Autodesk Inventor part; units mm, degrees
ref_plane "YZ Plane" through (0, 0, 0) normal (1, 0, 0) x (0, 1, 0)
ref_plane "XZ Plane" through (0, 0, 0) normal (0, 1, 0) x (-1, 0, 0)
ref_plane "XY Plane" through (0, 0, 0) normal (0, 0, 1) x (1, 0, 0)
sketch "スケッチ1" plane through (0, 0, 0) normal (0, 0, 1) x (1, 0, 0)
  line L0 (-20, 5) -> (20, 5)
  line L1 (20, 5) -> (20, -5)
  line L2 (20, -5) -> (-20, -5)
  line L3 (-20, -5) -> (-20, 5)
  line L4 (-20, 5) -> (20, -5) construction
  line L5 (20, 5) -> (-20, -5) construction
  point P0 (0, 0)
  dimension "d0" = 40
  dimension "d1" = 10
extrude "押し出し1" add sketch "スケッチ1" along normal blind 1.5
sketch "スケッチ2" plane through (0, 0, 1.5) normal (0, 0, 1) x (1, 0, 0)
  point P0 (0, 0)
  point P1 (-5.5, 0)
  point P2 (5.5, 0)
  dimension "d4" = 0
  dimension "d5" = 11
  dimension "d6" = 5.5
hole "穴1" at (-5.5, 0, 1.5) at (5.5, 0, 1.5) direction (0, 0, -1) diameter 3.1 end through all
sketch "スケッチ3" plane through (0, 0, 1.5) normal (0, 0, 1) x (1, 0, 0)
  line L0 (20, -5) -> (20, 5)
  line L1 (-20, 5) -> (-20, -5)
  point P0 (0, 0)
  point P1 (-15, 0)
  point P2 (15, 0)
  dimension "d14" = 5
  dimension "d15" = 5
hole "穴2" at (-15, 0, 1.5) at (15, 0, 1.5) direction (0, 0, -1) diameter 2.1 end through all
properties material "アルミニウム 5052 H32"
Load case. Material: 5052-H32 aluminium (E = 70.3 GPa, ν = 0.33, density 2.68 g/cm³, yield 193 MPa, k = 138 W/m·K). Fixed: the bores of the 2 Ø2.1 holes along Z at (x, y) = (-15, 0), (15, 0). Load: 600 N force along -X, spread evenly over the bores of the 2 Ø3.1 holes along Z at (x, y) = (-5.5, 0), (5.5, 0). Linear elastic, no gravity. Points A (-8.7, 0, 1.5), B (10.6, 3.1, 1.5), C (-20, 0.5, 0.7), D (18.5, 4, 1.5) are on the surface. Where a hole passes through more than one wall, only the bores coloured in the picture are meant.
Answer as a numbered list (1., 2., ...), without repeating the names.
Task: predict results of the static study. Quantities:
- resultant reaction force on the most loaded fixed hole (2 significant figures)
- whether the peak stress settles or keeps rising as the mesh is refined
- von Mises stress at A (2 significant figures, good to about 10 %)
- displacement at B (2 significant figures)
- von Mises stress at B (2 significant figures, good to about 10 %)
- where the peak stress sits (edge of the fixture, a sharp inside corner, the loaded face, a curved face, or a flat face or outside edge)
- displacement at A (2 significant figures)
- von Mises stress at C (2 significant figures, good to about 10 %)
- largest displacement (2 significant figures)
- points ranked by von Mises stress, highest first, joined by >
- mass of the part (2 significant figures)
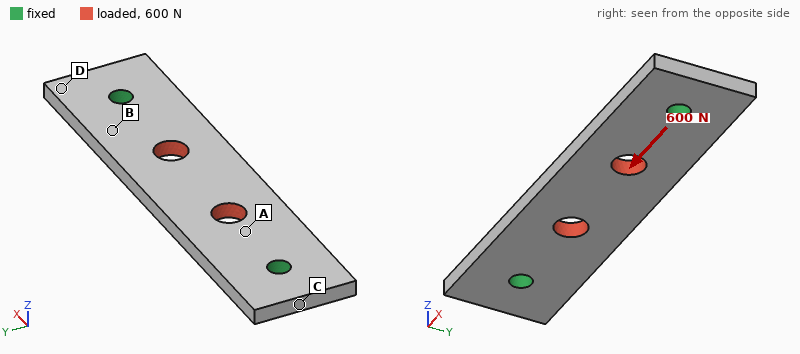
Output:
1. 300 N
2. keeps rising
3. 26 MPa
4. 2.0 µm
5. 19 MPa
6. edge of the fixture
7. 2.4 µm
8. 12 MPa
9. 4.6 µm
10. A > B > C > D
11. 1.5 g
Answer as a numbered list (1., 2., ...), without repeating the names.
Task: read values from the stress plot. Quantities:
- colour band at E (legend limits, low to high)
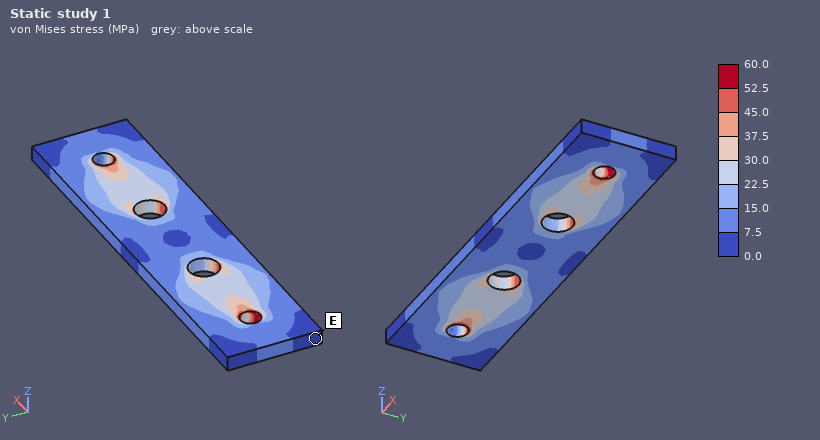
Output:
1. 0.0 to 7.5 MPa
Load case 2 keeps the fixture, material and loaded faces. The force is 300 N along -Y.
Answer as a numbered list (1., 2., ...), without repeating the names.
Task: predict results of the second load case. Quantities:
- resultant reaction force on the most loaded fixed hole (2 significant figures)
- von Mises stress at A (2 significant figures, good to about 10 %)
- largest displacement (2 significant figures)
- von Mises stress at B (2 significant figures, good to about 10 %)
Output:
1. 150 N
2. 31 MPa
3. 14 µm
4. 16 MPa
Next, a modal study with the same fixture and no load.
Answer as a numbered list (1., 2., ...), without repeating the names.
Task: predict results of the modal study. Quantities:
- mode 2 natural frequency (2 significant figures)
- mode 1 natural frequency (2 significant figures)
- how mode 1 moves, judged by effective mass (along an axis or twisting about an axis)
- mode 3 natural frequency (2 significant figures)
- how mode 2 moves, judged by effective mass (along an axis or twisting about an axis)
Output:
1. 15 kHz
2. 9000 Hz
3. along Z
4. 23 kHz
5. twisting about X
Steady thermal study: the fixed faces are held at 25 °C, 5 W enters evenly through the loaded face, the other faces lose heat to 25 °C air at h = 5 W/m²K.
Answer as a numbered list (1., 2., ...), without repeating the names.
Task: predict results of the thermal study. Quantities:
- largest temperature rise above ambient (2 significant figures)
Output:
1. 14 K
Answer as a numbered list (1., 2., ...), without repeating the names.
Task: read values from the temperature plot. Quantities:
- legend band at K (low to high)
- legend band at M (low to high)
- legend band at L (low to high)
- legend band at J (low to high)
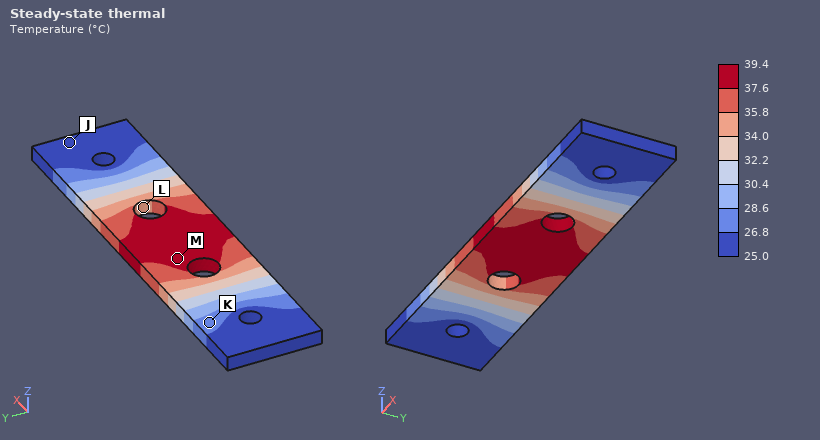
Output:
1. 26.8 to 28.6 °C
2. 37.6 to 39.4 °C
3. 34.0 to 35.8 °C
4. 25.0 to 26.8 °C
